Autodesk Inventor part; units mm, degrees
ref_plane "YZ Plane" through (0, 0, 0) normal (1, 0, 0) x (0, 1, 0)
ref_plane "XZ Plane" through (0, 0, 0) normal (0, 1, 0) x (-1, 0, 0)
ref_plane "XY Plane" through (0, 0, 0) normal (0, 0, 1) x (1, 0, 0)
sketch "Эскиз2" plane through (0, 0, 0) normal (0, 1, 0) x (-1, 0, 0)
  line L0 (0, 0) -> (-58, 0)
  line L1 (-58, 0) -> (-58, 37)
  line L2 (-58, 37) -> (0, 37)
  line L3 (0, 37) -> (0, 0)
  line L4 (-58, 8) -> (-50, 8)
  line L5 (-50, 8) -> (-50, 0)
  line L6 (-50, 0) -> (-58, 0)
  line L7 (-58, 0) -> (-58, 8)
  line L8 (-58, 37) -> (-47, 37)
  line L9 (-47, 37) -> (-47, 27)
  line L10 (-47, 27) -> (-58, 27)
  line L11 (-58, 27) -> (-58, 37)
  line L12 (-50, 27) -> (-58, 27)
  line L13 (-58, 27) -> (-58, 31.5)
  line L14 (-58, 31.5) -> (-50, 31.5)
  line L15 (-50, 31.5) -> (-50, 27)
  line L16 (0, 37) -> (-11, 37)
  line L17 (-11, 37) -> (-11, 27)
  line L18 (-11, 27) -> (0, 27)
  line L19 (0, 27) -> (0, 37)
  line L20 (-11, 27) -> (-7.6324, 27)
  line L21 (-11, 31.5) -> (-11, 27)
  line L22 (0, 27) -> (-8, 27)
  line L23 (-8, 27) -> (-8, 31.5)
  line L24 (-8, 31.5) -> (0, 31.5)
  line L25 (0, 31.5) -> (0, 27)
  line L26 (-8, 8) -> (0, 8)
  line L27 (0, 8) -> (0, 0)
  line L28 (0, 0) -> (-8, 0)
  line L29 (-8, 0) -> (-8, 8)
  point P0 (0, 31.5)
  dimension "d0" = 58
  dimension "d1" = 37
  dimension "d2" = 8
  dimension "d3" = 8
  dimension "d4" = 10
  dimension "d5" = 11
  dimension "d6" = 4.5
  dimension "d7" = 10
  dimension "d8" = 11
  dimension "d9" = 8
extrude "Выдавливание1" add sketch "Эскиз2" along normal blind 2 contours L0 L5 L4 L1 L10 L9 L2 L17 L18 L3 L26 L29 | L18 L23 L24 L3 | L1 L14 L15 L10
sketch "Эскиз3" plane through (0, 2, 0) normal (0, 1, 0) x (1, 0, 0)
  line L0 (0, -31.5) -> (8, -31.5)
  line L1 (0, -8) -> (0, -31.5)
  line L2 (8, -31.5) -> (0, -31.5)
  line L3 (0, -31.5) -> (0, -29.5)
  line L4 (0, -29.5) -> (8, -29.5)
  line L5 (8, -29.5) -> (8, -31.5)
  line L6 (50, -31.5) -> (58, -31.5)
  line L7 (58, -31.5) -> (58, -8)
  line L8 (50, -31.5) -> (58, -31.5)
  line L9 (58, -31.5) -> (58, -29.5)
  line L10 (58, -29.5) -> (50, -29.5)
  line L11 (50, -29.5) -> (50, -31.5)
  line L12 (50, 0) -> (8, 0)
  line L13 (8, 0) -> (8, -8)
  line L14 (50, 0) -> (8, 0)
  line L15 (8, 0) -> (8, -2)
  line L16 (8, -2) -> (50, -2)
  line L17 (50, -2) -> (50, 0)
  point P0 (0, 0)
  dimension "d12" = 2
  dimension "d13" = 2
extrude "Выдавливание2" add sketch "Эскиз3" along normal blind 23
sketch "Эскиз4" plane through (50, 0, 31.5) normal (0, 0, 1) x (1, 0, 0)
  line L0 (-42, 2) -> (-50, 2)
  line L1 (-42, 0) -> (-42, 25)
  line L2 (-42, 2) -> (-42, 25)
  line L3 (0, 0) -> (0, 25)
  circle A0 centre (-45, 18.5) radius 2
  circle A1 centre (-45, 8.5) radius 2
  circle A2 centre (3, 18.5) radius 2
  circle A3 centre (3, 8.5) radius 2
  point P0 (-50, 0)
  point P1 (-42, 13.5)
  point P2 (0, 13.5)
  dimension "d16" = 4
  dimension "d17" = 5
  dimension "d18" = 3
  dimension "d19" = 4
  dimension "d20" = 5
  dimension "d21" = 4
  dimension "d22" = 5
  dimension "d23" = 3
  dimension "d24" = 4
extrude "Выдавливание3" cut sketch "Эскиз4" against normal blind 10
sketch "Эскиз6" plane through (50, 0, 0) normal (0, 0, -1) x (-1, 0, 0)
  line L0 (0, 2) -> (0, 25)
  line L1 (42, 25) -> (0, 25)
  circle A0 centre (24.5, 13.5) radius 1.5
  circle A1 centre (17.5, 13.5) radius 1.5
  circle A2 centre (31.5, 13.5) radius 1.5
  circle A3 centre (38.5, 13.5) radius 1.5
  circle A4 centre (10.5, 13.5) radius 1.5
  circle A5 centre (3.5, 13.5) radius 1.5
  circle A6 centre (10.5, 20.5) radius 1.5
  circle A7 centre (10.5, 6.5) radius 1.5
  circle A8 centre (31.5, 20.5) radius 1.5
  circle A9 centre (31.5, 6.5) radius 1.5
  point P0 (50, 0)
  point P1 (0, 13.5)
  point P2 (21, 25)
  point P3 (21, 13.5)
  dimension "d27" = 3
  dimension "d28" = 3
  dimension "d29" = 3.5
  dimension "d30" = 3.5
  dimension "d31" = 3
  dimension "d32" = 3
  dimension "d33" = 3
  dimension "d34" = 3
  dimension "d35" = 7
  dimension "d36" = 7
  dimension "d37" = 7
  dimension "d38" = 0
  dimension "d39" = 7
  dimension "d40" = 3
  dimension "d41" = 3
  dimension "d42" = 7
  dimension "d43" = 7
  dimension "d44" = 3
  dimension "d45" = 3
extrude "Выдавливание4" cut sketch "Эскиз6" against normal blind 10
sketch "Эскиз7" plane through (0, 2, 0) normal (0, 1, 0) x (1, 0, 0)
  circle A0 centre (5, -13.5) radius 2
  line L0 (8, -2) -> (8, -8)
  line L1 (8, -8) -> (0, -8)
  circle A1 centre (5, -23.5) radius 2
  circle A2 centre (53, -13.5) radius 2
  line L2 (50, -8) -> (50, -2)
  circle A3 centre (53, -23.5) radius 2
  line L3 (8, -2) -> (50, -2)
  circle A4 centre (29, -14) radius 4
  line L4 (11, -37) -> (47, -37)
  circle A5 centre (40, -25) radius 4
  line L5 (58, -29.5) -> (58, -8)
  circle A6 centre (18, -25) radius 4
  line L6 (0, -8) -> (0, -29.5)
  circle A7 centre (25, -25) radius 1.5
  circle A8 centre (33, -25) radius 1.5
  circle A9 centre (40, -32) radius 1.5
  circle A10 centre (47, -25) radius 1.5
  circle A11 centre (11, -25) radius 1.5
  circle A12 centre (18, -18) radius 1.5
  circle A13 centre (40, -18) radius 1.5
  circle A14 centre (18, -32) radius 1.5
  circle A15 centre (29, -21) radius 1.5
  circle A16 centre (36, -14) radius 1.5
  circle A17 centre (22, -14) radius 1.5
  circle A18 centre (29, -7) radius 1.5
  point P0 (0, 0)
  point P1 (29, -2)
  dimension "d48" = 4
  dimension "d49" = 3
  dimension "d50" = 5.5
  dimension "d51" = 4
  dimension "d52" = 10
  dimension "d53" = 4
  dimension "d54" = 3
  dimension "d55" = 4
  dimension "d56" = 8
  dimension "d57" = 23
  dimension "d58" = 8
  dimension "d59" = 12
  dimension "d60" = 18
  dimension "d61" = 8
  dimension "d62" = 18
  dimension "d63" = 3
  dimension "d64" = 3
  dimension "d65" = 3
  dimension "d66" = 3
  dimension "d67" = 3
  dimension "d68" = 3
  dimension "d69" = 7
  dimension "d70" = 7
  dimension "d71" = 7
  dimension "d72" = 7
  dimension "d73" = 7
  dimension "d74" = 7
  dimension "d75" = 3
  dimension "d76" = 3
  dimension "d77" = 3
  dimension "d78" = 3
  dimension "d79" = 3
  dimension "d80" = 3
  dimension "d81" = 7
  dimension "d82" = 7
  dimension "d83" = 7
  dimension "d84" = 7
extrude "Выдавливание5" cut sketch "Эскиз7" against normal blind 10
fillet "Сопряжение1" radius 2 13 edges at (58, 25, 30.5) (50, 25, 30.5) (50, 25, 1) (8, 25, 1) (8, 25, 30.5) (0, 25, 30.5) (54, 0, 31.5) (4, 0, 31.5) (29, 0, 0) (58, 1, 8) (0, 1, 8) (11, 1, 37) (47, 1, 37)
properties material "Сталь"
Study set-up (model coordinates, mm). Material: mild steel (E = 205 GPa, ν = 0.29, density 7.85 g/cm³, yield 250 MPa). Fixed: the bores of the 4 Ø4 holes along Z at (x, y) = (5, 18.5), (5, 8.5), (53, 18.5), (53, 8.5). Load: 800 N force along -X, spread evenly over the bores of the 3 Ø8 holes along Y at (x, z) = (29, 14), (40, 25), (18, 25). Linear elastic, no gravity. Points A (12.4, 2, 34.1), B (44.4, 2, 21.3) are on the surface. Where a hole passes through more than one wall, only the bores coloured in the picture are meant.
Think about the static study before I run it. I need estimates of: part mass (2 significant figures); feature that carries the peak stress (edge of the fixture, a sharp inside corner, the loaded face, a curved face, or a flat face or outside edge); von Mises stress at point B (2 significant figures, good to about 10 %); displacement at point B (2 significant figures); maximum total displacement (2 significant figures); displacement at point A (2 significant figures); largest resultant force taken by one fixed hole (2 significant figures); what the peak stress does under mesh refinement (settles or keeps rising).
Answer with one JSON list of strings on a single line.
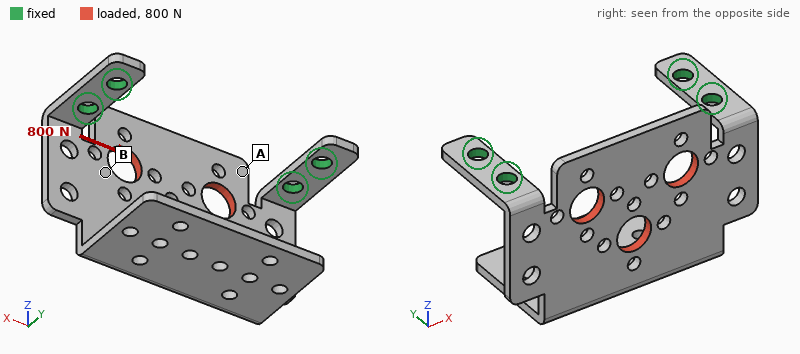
["43 g", "edge of the fixture", "41 MPa", "19 µm", "45 µm", "16 µm", "480 N", "keeps rising"]
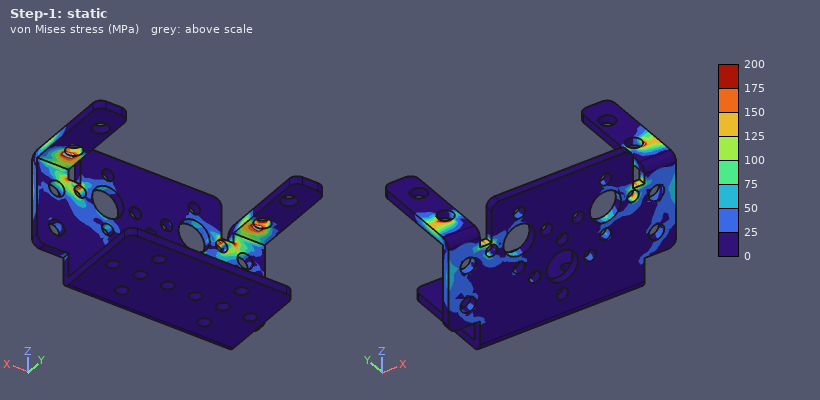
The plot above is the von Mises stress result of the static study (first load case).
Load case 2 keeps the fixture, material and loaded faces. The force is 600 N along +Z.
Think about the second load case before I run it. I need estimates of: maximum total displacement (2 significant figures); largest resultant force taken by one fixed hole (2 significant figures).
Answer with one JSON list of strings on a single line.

["0.18 mm", "310 N"]
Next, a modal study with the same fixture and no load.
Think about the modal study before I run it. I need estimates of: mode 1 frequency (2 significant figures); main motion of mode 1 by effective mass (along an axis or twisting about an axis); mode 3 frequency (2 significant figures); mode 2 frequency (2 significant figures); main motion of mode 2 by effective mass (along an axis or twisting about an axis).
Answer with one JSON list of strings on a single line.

["420 Hz", "along Y", "1700 Hz", "1300 Hz", "along X"]
